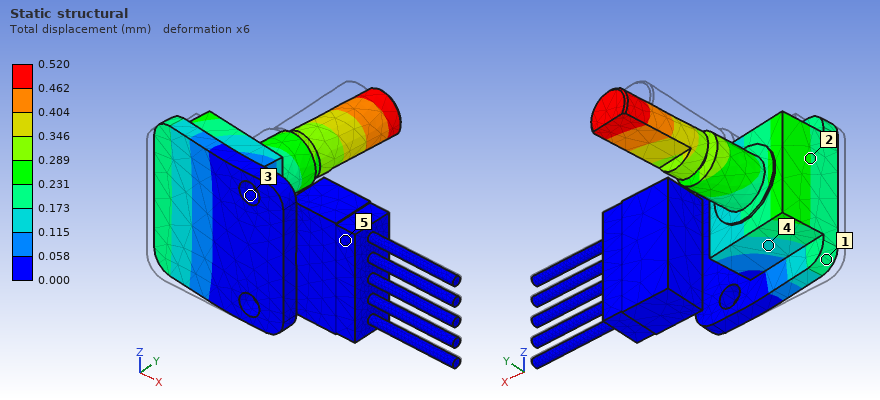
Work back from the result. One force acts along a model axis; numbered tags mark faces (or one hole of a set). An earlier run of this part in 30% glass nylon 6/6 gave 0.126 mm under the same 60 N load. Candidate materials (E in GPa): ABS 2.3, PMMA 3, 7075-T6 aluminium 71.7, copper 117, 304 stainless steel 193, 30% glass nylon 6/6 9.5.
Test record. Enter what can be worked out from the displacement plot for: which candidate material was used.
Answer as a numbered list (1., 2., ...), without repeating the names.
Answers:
1. ABS
